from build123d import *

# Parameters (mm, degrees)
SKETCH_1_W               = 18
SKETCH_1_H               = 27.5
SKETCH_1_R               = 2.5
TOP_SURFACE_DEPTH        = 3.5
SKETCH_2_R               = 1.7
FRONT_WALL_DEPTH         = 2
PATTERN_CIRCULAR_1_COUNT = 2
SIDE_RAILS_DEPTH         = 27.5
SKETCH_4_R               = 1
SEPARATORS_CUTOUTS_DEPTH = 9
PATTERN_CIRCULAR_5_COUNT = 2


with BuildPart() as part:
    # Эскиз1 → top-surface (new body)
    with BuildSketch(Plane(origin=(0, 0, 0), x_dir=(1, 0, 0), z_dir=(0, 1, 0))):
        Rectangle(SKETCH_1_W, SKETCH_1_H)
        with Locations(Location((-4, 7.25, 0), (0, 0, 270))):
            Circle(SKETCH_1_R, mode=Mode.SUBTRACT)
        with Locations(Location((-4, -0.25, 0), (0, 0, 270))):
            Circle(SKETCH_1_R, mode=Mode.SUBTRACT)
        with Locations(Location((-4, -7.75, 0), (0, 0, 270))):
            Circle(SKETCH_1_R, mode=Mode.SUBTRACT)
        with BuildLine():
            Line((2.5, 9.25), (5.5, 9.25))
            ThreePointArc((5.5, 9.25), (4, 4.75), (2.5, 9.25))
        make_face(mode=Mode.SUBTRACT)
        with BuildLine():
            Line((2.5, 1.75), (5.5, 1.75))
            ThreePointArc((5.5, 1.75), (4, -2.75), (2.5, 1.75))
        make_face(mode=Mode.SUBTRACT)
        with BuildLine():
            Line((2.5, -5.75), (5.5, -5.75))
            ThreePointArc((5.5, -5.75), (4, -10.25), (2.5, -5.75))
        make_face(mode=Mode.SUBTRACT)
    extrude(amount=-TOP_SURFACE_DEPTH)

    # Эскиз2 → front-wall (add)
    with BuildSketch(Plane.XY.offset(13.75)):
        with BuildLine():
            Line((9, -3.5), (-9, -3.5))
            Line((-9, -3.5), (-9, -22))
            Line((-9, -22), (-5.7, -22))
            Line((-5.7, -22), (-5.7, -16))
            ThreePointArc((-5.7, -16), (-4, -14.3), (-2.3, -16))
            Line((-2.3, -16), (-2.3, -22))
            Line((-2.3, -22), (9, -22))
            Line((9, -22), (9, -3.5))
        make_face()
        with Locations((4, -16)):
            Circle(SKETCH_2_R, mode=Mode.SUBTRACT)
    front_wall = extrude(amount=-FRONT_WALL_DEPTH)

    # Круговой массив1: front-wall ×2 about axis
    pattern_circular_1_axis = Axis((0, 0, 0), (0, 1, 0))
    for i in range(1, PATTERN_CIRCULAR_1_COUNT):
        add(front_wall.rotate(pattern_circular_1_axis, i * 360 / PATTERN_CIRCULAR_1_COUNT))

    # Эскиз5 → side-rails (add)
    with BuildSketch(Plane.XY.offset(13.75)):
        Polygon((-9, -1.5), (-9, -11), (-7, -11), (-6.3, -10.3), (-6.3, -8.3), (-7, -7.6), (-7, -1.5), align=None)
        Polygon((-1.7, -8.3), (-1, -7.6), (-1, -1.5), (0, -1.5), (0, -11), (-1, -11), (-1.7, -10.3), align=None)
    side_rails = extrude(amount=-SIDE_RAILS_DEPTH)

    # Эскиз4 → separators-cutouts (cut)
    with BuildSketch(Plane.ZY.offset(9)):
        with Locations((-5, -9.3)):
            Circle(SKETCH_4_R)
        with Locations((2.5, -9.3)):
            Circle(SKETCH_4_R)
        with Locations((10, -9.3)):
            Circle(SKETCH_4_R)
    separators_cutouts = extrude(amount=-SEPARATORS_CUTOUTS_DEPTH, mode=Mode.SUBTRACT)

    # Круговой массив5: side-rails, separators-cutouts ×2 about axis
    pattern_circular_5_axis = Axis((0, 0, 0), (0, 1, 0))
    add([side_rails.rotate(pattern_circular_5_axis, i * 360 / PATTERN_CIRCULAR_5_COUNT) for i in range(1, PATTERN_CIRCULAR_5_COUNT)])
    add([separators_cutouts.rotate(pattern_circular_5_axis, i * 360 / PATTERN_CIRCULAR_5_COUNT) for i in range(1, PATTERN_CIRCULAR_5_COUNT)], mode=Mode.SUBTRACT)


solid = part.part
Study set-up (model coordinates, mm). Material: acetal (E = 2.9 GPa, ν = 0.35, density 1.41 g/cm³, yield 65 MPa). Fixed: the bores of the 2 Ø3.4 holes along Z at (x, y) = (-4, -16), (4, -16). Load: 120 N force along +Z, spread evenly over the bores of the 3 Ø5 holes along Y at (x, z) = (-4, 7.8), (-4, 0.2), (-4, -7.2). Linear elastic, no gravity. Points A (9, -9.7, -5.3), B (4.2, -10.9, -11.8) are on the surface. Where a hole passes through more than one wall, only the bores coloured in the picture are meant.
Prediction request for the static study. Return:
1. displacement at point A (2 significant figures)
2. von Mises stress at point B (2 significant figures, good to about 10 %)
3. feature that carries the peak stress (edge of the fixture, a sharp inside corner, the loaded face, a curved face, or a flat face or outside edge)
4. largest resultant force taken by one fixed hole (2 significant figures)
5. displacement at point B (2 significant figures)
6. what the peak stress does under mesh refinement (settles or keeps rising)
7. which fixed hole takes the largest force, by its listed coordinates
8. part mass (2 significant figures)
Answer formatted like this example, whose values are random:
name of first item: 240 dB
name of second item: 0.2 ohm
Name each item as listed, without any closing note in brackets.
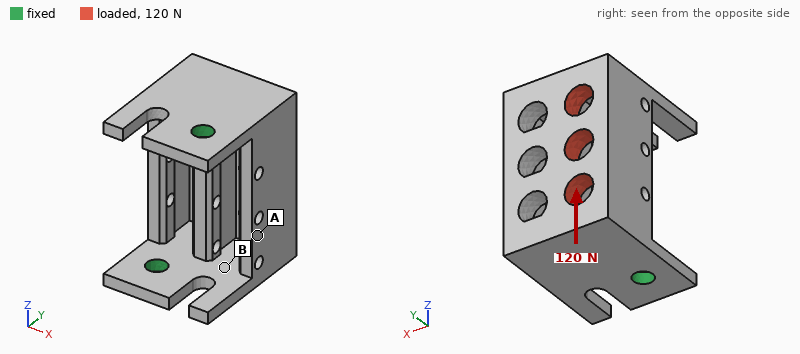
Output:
displacement at point A: 0.084 mm
von Mises stress at point B: 5.1 MPa
feature that carries the peak stress: edge of the fixture
largest resultant force taken by one fixed hole: 85 N
displacement at point B: 0.076 mm
what the peak stress does under mesh refinement: keeps rising
which fixed hole takes the largest force, by its listed coordinates: (-4, -16)
part mass: 5.2 g
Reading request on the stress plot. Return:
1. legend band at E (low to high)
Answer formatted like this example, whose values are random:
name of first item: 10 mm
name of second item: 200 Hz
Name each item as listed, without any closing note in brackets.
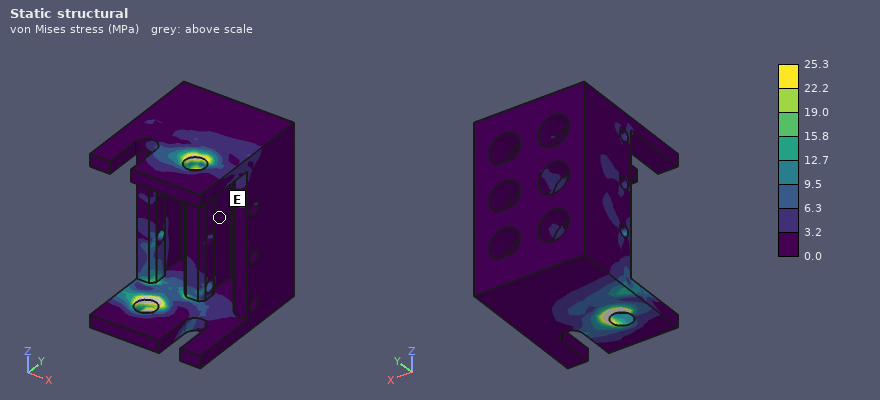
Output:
legend band at E: 0.0 to 3.2 MPa
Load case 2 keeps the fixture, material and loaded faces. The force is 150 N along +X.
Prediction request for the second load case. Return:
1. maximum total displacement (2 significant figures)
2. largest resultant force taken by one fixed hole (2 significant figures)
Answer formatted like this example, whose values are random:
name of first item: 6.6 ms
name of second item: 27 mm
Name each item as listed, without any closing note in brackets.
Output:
maximum total displacement: 0.39 mm
largest resultant force taken by one fixed hole: 76 N
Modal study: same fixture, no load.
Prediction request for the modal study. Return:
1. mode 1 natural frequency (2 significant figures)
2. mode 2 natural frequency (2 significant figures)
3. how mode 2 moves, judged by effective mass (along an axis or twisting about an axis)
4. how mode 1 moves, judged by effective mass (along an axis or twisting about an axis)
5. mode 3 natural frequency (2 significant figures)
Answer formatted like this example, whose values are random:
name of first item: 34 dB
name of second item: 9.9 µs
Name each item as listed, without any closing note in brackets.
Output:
mode 1 natural frequency: 1900 Hz
mode 2 natural frequency: 2900 Hz
how mode 2 moves, judged by effective mass: along Z
how mode 1 moves, judged by effective mass: along X
mode 3 natural frequency: 3200 Hz
